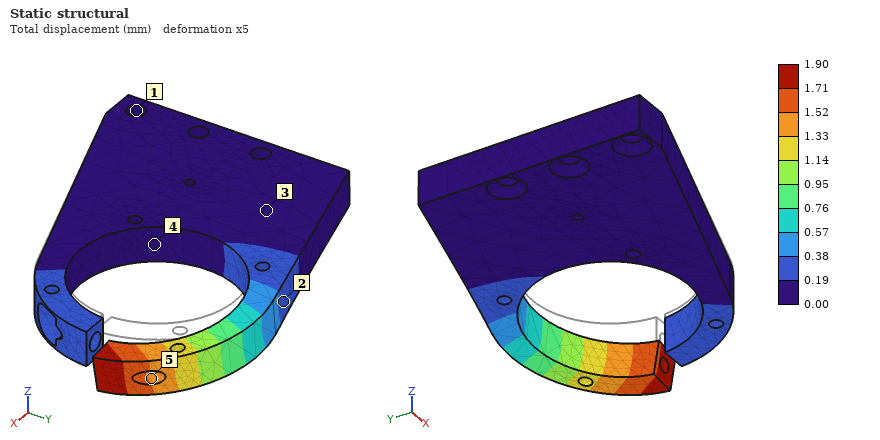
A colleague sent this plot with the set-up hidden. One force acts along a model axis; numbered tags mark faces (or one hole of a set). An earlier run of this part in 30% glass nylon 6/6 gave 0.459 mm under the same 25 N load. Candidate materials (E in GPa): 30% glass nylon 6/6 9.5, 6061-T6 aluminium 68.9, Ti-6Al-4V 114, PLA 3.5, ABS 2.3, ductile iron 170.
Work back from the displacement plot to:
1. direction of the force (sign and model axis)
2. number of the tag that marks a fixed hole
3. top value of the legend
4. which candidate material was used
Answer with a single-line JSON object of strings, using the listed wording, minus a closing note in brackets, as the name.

{"direction of the force": "-Z", "number of the tag that marks a fixed hole": "1", "top value of the legend": "1.90 mm", "which candidate material was used": "ABS"}
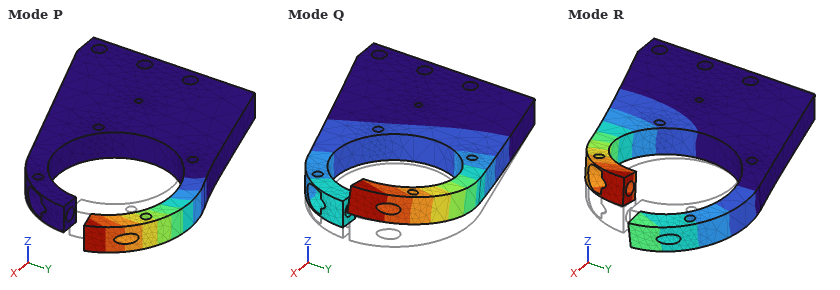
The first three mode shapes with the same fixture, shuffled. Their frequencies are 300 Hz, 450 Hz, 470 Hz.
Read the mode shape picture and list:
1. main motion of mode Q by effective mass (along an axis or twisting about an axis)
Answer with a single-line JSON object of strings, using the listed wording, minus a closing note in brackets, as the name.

{"main motion of mode Q by effective mass": "along Z"}
